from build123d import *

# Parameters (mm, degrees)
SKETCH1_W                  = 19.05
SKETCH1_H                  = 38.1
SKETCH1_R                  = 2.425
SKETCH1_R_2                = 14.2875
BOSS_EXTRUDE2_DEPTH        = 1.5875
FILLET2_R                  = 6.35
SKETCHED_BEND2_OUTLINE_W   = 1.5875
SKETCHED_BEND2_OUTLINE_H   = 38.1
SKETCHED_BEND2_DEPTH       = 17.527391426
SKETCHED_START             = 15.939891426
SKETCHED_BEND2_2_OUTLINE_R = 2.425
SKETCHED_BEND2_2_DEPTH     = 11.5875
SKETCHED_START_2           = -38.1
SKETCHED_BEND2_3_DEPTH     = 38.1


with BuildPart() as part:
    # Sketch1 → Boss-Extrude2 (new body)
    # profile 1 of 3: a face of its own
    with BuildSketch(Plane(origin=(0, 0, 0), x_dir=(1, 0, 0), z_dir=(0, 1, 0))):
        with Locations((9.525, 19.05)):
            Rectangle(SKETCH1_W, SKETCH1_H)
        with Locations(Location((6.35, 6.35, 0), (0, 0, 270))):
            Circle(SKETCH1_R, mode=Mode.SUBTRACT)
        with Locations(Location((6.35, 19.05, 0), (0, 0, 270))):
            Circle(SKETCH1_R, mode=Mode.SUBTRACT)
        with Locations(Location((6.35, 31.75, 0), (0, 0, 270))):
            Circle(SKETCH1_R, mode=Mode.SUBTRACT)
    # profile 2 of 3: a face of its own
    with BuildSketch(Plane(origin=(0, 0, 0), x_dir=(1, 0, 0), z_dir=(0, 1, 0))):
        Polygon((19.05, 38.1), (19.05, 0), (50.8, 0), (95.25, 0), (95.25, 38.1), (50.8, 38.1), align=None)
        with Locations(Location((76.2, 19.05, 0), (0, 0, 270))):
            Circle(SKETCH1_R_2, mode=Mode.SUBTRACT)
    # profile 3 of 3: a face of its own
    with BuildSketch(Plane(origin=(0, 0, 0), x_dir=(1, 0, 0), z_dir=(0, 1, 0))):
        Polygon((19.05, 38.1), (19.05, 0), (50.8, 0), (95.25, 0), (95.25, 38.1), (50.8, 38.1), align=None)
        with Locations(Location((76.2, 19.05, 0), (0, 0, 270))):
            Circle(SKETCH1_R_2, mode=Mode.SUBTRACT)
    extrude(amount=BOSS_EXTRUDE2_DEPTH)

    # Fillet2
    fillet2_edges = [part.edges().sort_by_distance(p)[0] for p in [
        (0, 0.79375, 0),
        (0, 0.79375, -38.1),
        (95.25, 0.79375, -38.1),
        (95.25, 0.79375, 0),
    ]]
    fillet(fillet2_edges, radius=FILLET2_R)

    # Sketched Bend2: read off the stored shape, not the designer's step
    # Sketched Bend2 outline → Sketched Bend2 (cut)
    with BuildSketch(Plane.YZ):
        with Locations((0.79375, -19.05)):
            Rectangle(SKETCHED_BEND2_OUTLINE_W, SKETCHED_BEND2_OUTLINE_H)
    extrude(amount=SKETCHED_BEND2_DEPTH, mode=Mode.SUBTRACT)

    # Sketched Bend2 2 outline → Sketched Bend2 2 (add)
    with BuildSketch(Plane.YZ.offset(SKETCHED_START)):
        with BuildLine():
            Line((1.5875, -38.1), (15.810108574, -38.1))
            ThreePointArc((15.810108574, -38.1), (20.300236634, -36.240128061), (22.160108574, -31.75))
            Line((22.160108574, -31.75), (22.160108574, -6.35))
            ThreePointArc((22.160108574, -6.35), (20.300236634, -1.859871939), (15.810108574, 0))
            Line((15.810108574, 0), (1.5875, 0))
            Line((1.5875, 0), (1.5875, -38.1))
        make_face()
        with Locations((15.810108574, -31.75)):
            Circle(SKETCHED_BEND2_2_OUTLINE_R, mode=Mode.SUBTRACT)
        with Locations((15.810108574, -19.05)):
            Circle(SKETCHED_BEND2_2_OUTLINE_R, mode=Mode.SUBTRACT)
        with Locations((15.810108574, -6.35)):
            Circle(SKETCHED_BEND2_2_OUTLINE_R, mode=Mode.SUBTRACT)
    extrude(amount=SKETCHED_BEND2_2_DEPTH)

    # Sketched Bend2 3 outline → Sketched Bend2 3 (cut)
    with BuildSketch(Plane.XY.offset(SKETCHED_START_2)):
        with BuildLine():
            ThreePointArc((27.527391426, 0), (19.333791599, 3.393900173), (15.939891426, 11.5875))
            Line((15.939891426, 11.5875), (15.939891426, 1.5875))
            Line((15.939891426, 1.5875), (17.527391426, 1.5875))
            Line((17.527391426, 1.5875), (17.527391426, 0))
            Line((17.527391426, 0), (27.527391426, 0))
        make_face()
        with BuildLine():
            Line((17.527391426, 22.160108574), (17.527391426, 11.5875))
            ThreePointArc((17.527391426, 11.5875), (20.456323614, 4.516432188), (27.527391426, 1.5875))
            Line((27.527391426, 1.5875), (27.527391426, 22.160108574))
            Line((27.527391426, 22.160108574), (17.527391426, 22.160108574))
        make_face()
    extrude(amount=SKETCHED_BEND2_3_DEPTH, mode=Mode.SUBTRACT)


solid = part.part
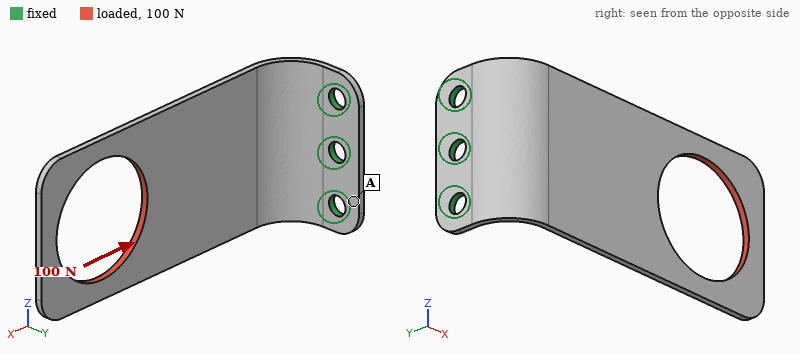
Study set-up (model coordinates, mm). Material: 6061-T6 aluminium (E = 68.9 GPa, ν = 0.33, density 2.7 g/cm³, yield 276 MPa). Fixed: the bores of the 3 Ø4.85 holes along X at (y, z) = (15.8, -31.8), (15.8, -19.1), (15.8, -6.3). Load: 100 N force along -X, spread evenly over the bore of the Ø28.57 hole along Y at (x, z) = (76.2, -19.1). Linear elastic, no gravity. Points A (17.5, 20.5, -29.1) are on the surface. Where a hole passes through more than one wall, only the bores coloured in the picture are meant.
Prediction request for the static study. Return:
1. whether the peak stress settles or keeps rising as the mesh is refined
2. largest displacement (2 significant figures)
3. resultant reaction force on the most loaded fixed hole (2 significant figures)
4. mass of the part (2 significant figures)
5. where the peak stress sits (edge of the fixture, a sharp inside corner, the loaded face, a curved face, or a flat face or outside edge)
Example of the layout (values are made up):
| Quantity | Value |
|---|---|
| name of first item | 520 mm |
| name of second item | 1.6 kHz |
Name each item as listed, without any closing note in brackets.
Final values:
| Quantity | Value |
|---|---|
| whether the peak stress settles or keeps rising as the mesh is refined | keeps rising |
| largest displacement | 0.81 mm |
| resultant reaction force on the most loaded fixed hole | 34 N |
| mass of the part | 12 g |
| where the peak stress sits | edge of the fixture |
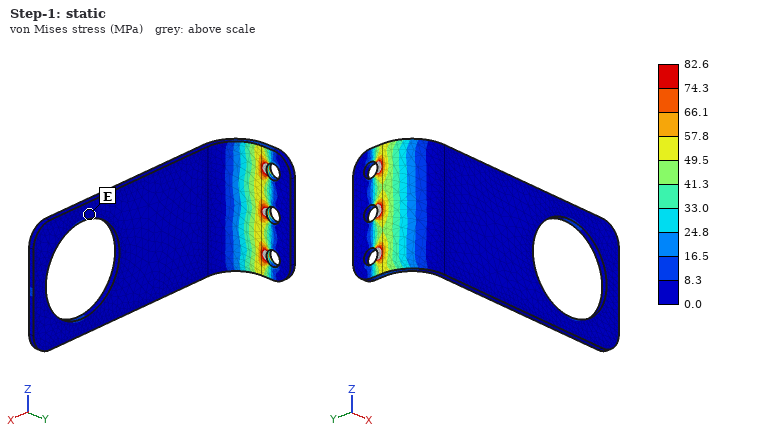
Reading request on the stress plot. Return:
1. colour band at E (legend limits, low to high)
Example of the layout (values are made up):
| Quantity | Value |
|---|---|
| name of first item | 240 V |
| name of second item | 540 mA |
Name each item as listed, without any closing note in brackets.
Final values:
| Quantity | Value |
|---|---|
| colour band at E | 0.0 to 8.3 MPa |
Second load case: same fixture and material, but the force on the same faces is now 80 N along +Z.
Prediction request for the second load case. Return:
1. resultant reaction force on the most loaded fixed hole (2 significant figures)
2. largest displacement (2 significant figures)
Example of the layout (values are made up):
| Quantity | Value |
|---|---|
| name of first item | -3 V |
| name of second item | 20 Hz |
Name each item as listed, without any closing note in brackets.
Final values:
| Quantity | Value |
|---|---|
| resultant reaction force on the most loaded fixed hole | 180 N |
| largest displacement | 0.97 mm |
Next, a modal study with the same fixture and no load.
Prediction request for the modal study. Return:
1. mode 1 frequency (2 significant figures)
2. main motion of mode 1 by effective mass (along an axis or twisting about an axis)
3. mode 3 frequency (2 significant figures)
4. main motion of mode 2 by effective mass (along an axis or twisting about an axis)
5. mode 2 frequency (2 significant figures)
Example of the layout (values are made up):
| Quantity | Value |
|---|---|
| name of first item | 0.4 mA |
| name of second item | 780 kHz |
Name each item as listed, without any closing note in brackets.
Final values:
| Quantity | Value |
|---|---|
| mode 1 frequency | 230 Hz |
| main motion of mode 1 by effective mass | along Y |
| mode 3 frequency | 990 Hz |
| main motion of mode 2 by effective mass | along Z |
| mode 2 frequency | 710 Hz |
